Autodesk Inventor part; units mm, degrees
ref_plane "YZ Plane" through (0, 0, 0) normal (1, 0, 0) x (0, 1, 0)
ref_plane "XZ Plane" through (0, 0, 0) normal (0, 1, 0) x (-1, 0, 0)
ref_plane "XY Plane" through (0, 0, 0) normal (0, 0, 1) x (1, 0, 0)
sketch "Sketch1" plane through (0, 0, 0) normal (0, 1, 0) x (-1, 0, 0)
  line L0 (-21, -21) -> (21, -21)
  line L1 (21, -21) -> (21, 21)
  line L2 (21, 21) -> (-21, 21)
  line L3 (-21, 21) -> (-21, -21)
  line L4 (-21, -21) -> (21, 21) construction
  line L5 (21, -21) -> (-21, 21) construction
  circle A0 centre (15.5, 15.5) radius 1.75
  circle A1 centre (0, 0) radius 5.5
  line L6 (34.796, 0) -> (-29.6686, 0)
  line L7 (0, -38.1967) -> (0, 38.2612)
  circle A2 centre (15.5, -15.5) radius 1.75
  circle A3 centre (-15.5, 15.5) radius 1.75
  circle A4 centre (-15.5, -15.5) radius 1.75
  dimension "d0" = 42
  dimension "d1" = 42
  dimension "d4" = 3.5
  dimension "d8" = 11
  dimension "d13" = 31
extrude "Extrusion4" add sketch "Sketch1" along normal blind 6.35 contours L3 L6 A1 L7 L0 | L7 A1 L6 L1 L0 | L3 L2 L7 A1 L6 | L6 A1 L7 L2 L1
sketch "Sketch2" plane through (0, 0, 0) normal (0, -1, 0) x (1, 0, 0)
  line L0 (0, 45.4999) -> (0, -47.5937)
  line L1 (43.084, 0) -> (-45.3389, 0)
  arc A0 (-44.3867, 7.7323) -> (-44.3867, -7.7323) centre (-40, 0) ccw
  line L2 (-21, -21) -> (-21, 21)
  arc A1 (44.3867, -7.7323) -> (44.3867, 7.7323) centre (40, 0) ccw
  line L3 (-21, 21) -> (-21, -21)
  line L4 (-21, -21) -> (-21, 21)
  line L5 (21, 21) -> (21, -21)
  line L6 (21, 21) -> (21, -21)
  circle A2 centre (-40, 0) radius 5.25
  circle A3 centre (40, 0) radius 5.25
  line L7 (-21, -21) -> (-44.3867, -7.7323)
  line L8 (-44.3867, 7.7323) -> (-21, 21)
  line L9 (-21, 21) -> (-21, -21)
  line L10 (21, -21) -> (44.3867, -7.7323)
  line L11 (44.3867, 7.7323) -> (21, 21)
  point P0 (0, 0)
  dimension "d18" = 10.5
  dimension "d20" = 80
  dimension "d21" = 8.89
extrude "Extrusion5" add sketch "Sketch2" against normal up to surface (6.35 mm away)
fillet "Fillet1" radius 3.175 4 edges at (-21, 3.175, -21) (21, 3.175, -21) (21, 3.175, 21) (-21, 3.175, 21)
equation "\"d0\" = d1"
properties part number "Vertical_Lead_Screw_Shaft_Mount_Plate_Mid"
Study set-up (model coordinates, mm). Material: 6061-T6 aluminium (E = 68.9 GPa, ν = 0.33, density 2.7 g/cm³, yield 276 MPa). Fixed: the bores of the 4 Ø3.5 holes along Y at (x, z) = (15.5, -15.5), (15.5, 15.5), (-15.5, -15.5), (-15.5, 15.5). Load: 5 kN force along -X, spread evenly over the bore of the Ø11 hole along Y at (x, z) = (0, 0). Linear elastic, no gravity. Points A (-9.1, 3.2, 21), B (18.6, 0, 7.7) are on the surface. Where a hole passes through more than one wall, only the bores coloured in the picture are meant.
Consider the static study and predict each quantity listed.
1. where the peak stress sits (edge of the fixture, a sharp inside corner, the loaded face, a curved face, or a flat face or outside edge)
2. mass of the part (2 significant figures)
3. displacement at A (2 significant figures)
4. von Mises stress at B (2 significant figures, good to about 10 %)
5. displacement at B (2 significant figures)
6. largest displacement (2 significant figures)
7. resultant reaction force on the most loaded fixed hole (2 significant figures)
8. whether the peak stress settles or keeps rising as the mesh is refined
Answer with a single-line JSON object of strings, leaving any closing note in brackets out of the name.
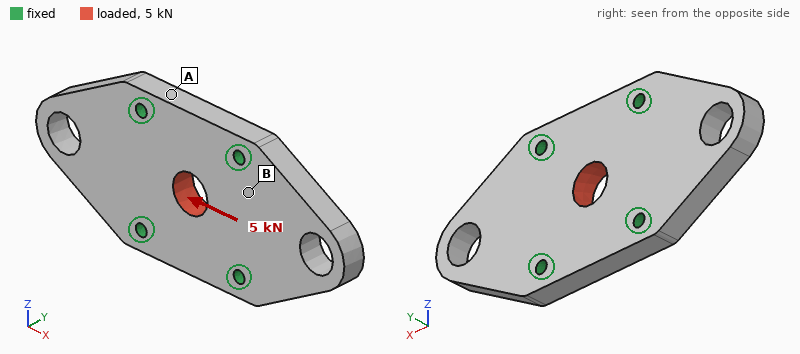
{"where the peak stress sits": "edge of the fixture", "mass of the part": "50 g", "displacement at A": "0.87 µm", "von Mises stress at B": "8.7 MPa", "displacement at B": "2.2 µm", "largest displacement": "5.7 µm", "resultant reaction force on the most loaded fixed hole": "1.3 kN", "whether the peak stress settles or keeps rising as the mesh is refined": "keeps rising"}
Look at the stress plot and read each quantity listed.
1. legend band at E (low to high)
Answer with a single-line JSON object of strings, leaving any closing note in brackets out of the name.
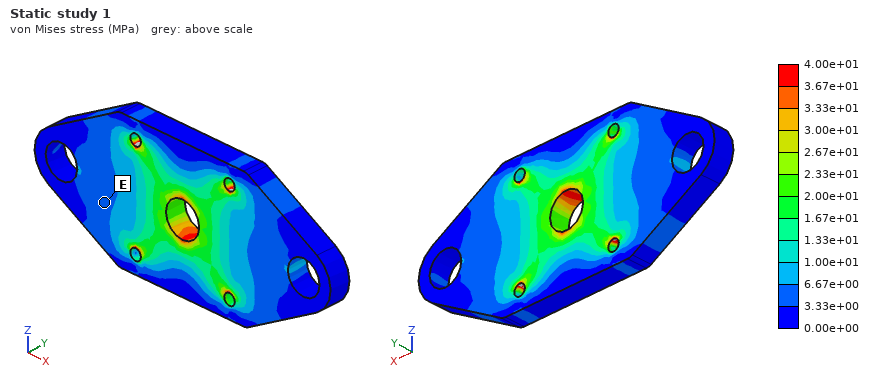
{"legend band at E": "3.33e+00 to 6.67e+00 MPa"}
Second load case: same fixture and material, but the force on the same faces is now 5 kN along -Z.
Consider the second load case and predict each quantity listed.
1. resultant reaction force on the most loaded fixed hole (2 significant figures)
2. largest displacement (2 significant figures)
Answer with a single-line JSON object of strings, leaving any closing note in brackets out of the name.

{"resultant reaction force on the most loaded fixed hole": "1.4 kN", "largest displacement": "7.1 µm"}
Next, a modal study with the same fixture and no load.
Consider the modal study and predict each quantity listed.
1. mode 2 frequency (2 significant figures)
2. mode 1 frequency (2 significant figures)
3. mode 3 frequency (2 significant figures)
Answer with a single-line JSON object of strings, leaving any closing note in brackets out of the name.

{"mode 2 frequency": "6700 Hz", "mode 1 frequency": "6600 Hz", "mode 3 frequency": "18 kHz"}
